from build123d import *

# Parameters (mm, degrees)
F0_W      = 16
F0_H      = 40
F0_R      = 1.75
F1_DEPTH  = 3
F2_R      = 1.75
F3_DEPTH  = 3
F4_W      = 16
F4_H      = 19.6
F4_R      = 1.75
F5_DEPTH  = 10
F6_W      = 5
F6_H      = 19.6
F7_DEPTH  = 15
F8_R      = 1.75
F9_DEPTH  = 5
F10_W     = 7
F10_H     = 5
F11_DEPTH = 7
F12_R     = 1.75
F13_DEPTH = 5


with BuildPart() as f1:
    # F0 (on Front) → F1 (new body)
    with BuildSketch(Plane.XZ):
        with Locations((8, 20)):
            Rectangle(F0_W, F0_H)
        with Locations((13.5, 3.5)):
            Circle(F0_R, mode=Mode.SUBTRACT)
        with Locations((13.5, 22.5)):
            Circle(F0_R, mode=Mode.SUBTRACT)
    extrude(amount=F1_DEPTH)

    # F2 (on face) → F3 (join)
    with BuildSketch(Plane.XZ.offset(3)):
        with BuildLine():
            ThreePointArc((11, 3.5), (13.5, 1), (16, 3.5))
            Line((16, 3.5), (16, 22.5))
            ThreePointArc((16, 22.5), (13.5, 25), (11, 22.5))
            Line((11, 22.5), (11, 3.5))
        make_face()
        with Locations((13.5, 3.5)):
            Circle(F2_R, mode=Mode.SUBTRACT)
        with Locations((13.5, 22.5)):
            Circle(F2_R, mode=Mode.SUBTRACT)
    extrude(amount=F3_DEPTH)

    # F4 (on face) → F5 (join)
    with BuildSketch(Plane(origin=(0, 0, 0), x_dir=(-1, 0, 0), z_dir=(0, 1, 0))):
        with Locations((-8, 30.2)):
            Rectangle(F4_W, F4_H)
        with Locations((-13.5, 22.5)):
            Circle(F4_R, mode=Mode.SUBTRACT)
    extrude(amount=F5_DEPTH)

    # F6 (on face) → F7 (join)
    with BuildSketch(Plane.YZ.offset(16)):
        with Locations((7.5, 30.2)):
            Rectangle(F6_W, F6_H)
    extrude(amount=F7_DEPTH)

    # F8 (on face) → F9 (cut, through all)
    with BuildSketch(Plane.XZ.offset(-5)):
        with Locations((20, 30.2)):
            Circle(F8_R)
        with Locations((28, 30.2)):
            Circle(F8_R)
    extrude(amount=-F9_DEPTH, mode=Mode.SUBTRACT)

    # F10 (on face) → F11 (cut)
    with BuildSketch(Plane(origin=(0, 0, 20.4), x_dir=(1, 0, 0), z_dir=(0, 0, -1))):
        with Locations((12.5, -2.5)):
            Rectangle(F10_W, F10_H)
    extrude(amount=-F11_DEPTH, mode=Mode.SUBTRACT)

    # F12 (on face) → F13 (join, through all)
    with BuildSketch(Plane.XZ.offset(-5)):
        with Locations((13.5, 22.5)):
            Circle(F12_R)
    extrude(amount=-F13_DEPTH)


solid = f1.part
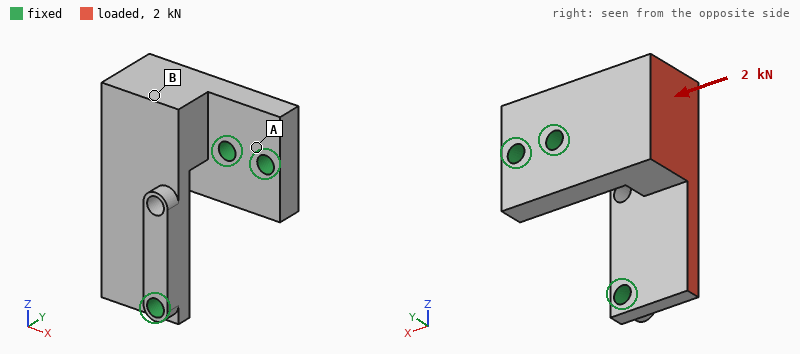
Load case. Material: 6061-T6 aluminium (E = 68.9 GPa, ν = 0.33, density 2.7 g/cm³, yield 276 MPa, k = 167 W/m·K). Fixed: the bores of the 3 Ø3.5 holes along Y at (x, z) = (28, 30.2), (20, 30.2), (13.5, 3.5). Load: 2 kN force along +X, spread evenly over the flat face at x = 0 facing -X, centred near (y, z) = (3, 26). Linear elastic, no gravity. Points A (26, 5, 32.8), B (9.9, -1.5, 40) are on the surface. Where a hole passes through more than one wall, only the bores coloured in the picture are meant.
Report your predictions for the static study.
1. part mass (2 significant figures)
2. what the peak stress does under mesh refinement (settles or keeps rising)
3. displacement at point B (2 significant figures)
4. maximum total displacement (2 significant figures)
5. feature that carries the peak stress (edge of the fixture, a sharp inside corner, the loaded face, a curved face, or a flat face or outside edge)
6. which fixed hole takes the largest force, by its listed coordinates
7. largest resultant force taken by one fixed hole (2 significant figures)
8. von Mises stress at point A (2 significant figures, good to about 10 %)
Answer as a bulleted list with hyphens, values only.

- 17 g
- keeps rising
- 29 µm
- 45 µm
- edge of the fixture
- (20, 30.2)
- 1.3 kN
- 20 MPa
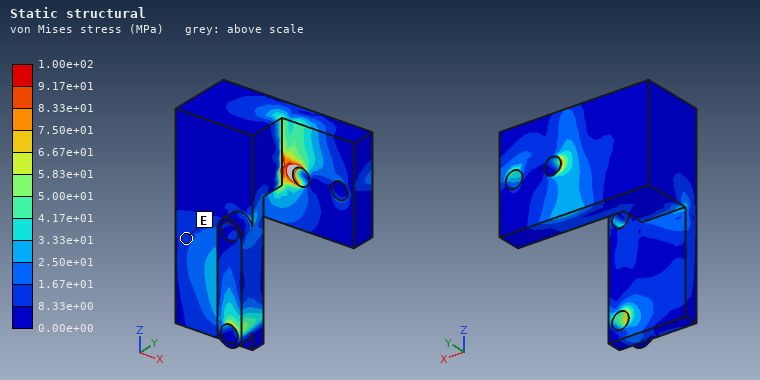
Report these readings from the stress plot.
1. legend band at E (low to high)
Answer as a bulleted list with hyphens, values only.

- 8.33e+00 to 1.67e+01 MPa
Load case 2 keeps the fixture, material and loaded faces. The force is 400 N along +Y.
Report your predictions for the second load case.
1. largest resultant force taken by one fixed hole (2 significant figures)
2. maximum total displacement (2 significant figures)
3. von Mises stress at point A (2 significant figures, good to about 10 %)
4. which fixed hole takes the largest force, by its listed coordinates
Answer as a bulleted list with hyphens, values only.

- 590 N
- 40 µm
- 10 MPa
- (20, 30.2)
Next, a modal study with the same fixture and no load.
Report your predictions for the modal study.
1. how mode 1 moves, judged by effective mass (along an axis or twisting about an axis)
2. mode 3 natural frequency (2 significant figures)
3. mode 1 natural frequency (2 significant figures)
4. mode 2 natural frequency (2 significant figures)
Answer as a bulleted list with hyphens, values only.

- along Y
- 21 kHz
- 7200 Hz
- 16 kHz
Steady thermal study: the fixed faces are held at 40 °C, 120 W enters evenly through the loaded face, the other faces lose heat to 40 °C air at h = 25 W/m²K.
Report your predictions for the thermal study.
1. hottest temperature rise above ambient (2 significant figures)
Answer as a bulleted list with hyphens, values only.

- 73 K
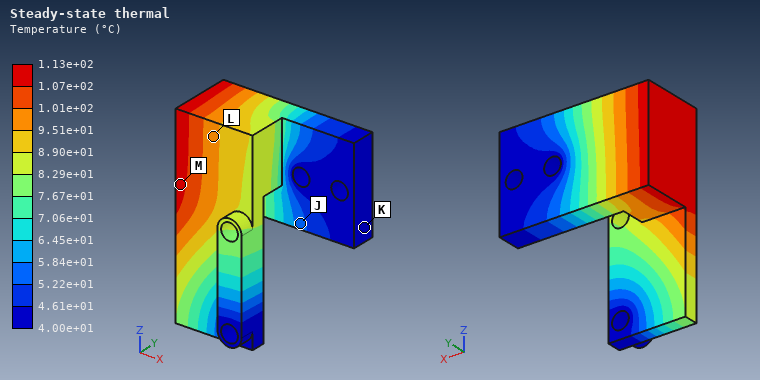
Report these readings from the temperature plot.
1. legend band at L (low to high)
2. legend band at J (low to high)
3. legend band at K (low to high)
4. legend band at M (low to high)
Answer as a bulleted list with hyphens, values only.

- 9.51e+01 to 1.01e+02 °C
- 5.22e+01 to 5.84e+01 °C
- 4.00e+01 to 4.61e+01 °C
- 1.07e+02 to 1.13e+02 °C
